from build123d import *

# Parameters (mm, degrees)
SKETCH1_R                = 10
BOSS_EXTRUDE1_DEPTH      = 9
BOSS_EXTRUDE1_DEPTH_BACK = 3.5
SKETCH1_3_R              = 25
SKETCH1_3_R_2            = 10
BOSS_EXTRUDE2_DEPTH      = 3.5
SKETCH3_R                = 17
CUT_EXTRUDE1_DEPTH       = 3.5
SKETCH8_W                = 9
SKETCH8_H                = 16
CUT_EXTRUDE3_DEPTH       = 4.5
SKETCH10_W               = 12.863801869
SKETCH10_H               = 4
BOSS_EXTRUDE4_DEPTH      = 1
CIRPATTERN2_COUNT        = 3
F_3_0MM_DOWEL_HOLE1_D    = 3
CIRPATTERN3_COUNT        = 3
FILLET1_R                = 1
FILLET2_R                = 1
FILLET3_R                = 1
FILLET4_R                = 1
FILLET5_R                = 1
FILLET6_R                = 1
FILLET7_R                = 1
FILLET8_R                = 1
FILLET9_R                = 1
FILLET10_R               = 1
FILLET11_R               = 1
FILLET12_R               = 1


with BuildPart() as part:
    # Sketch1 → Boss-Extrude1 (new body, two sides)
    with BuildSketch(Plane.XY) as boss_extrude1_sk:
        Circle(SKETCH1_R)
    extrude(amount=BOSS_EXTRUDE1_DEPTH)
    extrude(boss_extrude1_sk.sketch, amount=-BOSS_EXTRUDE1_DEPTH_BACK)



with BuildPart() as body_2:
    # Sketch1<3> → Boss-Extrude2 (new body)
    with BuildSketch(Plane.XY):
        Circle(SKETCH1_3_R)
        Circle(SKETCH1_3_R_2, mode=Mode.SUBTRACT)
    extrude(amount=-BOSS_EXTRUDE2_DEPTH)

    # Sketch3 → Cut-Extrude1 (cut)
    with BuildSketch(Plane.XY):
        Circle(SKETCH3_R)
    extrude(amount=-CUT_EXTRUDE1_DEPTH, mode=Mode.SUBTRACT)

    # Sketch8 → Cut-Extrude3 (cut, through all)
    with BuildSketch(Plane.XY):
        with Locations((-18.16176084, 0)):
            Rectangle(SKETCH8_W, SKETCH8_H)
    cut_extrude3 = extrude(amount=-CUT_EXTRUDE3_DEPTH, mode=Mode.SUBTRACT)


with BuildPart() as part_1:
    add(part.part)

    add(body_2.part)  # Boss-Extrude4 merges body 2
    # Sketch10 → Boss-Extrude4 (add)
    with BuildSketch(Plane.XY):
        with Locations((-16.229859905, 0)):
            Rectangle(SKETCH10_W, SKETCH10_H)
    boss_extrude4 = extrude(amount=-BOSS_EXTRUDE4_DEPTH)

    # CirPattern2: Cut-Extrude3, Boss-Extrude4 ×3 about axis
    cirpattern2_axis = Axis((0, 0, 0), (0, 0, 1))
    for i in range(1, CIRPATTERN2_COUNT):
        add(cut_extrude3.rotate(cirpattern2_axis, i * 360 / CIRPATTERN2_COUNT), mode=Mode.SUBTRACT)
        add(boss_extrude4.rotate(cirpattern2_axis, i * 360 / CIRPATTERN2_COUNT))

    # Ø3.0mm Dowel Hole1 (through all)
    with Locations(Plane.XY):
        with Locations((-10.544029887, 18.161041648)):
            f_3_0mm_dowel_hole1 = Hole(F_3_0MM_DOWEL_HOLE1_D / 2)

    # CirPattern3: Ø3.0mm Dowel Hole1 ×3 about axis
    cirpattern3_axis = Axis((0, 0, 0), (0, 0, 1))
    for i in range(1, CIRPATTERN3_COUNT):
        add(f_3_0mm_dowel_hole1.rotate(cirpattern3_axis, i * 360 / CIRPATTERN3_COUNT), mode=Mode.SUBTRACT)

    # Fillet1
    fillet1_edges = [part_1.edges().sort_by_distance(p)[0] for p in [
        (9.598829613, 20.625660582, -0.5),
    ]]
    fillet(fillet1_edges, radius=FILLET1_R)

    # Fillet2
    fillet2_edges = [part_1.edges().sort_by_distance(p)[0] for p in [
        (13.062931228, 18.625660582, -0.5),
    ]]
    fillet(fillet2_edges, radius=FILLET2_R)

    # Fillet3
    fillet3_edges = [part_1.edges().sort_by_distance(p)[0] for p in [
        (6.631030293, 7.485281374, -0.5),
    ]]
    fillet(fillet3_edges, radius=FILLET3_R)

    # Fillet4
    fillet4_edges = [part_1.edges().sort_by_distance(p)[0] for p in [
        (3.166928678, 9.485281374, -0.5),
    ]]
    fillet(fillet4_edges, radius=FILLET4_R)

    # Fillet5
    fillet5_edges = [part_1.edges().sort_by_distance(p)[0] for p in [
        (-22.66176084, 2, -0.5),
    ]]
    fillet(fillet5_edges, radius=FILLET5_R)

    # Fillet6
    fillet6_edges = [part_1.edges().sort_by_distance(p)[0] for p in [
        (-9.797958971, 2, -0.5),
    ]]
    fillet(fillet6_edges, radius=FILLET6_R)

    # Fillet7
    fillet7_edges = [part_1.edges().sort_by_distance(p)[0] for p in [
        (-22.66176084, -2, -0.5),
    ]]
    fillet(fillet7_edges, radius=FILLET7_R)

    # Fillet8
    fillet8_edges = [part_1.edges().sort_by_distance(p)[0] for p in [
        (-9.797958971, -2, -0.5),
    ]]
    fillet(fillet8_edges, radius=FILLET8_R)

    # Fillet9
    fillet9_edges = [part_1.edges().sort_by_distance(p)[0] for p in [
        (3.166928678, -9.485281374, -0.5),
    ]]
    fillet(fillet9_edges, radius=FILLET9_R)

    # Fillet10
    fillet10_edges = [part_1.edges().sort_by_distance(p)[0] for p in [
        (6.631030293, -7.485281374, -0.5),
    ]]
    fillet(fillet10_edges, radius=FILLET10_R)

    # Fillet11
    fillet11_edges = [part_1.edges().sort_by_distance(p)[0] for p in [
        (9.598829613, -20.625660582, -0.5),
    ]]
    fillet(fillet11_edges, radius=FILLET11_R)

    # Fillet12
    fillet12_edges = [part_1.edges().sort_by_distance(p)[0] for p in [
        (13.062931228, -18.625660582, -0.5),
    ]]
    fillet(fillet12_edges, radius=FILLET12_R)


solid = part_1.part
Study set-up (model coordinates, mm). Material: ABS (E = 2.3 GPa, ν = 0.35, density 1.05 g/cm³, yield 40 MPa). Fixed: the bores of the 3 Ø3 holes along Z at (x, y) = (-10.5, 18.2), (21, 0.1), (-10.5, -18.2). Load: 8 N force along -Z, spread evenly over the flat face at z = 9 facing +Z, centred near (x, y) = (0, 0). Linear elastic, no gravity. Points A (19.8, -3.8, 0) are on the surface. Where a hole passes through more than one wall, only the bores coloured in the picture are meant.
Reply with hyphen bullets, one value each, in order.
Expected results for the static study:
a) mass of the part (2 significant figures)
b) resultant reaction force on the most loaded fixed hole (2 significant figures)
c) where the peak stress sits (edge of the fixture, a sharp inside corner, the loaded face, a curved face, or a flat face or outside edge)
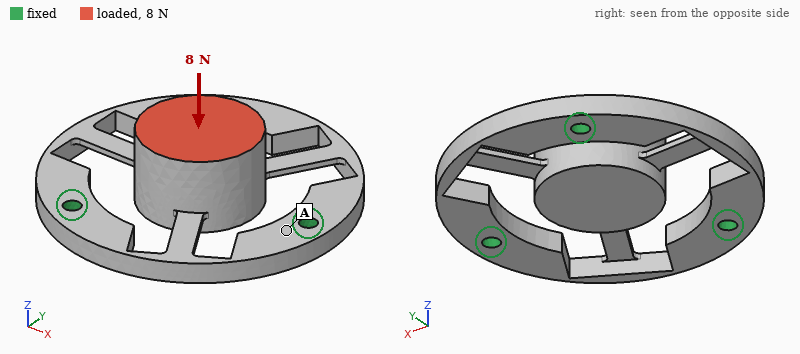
- 7.0 g
- 2.9 N
- a curved face
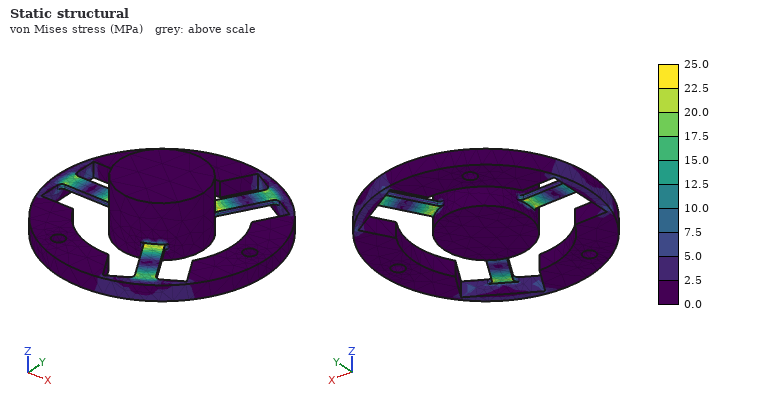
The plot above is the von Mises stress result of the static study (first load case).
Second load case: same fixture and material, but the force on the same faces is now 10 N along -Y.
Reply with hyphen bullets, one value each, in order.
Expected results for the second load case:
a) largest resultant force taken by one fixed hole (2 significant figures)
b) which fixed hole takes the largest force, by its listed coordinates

- 6.9 N
- (21, 0.1)
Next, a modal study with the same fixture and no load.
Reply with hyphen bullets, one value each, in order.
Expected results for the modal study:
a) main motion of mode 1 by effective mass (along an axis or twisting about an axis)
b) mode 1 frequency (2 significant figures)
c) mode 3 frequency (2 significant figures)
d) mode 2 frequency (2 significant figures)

- along Z
- 250 Hz
- 440 Hz
- 440 Hz
